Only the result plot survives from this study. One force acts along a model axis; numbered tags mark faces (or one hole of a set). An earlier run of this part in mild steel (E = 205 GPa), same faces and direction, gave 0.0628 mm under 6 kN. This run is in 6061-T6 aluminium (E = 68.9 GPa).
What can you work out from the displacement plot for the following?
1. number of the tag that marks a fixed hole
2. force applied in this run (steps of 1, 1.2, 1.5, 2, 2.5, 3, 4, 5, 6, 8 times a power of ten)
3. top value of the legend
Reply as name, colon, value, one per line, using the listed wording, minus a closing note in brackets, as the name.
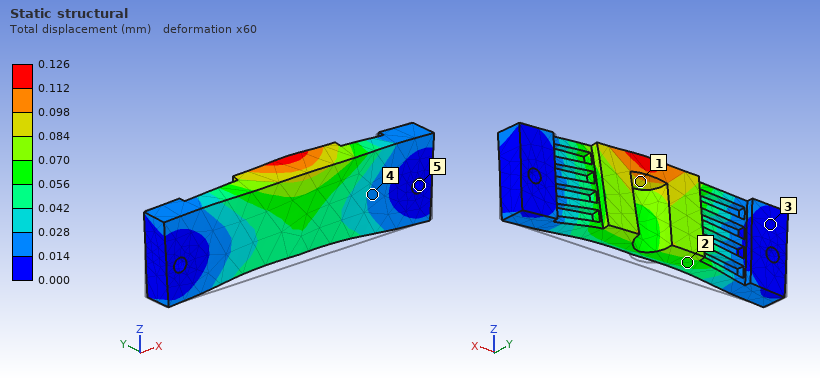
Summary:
number of the tag that marks a fixed hole: 5
force applied in this run: 4 kN
top value of the legend: 0.126 mm
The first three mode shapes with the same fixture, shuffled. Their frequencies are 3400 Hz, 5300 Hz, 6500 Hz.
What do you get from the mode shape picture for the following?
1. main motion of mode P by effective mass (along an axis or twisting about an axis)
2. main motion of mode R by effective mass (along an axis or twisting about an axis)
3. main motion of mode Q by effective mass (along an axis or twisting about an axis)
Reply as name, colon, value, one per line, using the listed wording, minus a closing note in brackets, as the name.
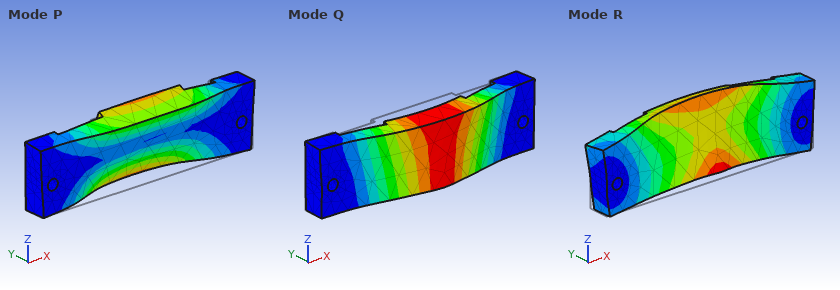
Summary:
main motion of mode P by effective mass: along Z
main motion of mode R by effective mass: along Z
main motion of mode Q by effective mass: along Y
